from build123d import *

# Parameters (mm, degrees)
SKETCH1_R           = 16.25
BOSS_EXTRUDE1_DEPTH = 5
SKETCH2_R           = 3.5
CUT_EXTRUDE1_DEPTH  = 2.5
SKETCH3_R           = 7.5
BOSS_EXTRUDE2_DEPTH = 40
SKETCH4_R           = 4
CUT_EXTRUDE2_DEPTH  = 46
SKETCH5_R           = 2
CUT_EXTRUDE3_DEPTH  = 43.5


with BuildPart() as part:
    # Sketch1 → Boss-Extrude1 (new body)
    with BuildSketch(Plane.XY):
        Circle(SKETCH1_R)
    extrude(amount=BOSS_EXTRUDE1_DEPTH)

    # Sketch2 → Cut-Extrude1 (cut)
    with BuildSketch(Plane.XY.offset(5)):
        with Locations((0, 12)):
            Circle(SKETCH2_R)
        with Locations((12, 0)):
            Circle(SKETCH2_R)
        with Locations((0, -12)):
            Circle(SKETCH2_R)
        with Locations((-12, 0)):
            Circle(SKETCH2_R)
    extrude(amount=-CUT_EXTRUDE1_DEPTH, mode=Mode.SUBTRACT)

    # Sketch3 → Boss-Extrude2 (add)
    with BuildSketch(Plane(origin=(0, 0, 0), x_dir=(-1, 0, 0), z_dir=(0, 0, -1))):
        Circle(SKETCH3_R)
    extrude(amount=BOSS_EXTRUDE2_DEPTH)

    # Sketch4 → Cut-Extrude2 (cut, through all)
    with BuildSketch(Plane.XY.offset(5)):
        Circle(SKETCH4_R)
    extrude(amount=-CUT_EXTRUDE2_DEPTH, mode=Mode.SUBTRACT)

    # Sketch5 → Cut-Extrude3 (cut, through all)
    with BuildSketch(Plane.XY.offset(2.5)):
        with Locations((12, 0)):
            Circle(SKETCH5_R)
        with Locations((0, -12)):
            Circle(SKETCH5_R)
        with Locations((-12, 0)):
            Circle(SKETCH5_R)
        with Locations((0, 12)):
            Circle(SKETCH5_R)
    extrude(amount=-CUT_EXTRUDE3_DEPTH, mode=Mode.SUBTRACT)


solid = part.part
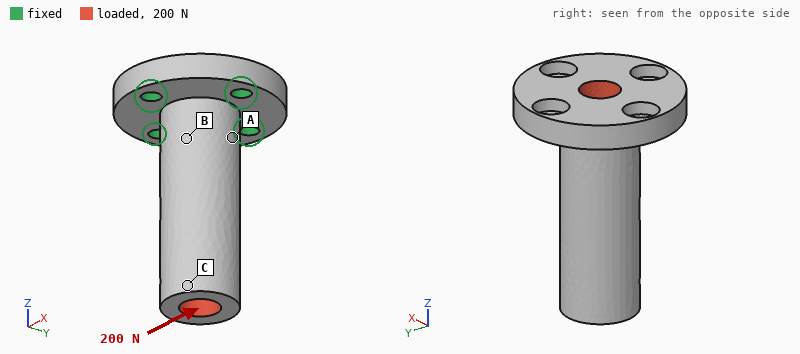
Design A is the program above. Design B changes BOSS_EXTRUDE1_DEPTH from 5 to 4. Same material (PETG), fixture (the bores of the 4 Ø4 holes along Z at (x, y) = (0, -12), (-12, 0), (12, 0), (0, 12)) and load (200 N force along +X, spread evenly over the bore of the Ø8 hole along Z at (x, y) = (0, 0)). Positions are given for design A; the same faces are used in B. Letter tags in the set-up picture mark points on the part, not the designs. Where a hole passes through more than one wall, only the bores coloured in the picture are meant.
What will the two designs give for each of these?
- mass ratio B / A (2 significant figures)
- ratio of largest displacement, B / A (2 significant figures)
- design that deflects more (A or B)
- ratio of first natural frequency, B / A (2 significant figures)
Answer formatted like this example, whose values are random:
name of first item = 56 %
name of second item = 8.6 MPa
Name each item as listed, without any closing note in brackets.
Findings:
mass ratio B / A = 0.93
ratio of largest displacement, B / A = 1.1
design that deflects more = B
ratio of first natural frequency, B / A = 0.96
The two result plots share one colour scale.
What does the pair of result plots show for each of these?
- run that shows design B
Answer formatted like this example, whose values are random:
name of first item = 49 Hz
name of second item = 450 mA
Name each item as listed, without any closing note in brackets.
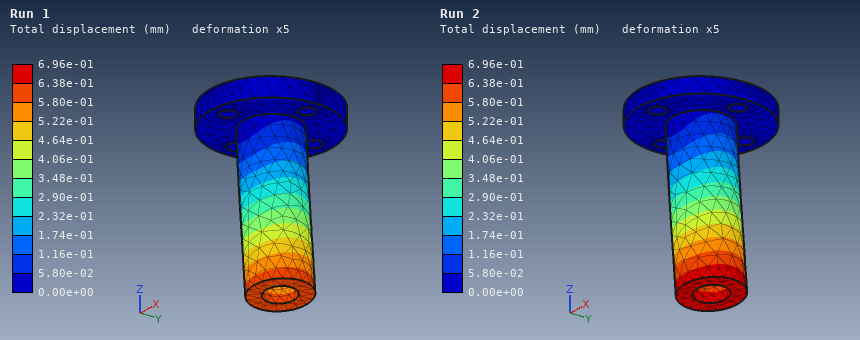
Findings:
run that shows design B = Run 2
